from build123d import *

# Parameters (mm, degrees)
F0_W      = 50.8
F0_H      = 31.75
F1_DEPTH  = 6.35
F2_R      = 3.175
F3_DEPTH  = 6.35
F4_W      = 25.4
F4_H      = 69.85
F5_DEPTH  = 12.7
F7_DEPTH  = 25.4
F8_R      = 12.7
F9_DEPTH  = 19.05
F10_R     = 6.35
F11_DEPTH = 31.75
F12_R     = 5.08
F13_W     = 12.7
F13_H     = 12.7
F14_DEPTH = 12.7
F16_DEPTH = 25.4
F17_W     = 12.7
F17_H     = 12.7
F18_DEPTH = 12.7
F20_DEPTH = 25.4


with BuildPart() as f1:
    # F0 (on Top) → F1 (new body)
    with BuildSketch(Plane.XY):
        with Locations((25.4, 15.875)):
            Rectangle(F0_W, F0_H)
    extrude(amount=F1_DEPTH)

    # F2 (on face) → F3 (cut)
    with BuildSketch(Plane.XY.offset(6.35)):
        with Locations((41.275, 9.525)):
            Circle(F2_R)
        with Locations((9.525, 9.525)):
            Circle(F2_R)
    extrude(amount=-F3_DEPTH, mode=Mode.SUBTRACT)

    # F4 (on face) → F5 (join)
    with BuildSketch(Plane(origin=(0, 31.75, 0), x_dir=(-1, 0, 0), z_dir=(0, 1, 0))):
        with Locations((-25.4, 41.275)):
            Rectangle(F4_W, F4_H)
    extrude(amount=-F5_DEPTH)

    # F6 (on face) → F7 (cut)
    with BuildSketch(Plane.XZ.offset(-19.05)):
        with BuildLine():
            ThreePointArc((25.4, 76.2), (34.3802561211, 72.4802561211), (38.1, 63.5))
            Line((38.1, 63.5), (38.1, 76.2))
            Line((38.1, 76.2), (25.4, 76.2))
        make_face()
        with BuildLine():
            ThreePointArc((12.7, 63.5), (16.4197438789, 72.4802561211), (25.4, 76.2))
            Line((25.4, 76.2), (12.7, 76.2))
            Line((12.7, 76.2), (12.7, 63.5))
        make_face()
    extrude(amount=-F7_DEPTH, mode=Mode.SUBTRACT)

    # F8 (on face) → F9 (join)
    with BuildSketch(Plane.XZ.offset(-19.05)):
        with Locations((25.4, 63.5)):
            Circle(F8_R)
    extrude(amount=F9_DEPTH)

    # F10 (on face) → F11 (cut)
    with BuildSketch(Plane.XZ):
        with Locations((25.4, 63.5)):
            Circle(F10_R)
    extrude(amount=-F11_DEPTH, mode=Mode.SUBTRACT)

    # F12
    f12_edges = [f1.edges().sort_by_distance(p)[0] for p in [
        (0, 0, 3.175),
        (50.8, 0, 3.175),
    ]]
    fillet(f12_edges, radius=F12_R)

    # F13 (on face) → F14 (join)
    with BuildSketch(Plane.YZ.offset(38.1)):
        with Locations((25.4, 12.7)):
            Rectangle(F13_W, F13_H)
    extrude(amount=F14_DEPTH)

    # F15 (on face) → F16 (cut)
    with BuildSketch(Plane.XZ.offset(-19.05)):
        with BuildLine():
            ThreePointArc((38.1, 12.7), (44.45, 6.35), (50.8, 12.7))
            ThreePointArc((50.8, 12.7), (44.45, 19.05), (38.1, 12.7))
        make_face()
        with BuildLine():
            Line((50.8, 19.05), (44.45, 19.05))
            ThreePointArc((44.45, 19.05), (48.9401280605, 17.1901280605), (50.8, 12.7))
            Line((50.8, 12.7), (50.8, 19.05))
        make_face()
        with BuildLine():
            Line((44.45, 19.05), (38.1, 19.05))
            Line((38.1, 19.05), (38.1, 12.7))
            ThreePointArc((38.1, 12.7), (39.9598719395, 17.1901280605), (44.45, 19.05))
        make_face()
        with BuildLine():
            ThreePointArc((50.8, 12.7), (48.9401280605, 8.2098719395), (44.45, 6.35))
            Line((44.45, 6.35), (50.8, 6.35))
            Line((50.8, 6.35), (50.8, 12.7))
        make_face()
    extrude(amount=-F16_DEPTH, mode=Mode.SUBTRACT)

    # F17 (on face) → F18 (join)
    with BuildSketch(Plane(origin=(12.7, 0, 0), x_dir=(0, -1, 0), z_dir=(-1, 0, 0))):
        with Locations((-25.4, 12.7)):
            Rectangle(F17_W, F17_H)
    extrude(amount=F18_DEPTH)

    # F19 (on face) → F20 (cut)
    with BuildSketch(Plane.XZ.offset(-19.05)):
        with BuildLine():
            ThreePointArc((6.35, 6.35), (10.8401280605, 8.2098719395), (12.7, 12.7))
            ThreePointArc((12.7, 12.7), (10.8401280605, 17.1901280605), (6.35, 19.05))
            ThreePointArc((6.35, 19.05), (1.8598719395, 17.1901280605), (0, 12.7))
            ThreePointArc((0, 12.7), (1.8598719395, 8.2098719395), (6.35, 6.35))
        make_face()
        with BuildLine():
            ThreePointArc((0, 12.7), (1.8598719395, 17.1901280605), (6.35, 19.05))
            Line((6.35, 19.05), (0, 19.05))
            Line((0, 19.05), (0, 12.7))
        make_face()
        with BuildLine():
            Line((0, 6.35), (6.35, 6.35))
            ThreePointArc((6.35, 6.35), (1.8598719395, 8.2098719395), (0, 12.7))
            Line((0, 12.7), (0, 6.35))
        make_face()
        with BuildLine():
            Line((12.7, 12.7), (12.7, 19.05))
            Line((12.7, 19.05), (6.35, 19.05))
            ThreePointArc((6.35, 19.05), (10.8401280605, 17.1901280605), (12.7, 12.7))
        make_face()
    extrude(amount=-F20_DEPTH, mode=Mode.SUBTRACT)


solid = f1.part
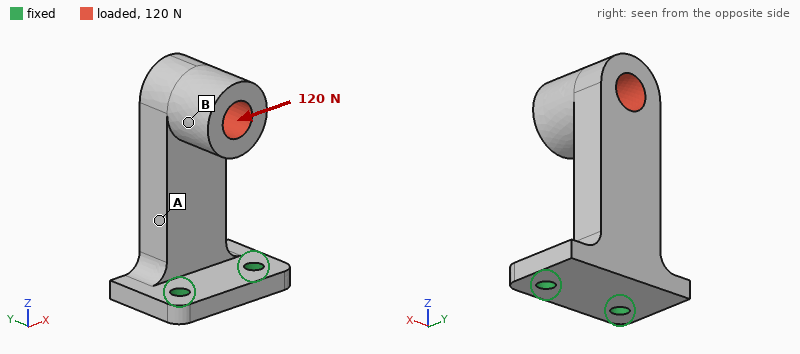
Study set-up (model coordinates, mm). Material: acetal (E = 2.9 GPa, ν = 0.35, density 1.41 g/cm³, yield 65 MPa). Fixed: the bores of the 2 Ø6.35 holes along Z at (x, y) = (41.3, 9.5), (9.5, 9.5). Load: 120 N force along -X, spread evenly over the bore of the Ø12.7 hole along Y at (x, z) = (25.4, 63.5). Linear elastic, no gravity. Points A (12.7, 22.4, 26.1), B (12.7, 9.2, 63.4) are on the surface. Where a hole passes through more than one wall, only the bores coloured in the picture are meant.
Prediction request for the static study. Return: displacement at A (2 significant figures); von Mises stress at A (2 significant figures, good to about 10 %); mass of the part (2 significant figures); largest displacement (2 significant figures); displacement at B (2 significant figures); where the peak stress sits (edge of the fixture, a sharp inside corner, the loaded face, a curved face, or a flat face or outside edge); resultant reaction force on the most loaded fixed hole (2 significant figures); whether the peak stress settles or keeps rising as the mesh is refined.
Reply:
0.19 mm
3.7 MPa
53 g
0.76 mm
0.60 mm
edge of the fixture
240 N
keeps rising
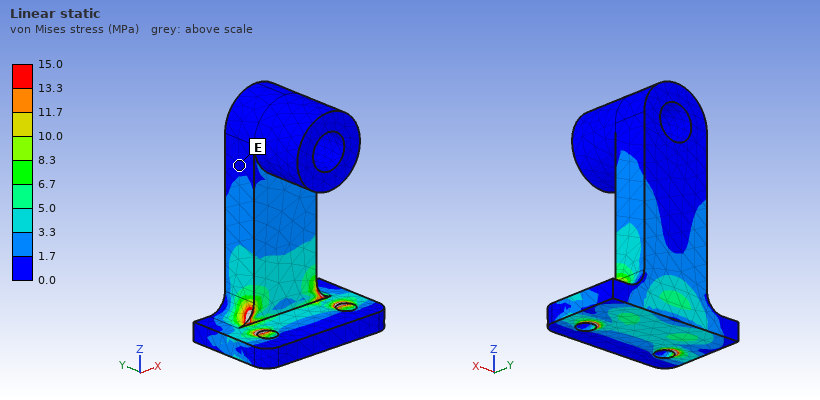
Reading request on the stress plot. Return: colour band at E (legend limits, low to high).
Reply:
0.0 to 1.7 MPa
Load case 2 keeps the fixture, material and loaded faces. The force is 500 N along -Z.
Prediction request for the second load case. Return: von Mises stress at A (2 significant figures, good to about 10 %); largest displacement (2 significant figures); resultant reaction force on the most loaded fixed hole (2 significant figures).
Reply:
4.8 MPa
1.1 mm
250 N
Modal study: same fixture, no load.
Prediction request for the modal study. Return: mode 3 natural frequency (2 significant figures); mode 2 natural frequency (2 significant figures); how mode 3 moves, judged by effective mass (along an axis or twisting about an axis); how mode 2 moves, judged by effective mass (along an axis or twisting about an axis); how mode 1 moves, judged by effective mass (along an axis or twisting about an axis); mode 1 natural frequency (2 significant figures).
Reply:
1200 Hz
510 Hz
along Z
along X
along Y
240 Hz
